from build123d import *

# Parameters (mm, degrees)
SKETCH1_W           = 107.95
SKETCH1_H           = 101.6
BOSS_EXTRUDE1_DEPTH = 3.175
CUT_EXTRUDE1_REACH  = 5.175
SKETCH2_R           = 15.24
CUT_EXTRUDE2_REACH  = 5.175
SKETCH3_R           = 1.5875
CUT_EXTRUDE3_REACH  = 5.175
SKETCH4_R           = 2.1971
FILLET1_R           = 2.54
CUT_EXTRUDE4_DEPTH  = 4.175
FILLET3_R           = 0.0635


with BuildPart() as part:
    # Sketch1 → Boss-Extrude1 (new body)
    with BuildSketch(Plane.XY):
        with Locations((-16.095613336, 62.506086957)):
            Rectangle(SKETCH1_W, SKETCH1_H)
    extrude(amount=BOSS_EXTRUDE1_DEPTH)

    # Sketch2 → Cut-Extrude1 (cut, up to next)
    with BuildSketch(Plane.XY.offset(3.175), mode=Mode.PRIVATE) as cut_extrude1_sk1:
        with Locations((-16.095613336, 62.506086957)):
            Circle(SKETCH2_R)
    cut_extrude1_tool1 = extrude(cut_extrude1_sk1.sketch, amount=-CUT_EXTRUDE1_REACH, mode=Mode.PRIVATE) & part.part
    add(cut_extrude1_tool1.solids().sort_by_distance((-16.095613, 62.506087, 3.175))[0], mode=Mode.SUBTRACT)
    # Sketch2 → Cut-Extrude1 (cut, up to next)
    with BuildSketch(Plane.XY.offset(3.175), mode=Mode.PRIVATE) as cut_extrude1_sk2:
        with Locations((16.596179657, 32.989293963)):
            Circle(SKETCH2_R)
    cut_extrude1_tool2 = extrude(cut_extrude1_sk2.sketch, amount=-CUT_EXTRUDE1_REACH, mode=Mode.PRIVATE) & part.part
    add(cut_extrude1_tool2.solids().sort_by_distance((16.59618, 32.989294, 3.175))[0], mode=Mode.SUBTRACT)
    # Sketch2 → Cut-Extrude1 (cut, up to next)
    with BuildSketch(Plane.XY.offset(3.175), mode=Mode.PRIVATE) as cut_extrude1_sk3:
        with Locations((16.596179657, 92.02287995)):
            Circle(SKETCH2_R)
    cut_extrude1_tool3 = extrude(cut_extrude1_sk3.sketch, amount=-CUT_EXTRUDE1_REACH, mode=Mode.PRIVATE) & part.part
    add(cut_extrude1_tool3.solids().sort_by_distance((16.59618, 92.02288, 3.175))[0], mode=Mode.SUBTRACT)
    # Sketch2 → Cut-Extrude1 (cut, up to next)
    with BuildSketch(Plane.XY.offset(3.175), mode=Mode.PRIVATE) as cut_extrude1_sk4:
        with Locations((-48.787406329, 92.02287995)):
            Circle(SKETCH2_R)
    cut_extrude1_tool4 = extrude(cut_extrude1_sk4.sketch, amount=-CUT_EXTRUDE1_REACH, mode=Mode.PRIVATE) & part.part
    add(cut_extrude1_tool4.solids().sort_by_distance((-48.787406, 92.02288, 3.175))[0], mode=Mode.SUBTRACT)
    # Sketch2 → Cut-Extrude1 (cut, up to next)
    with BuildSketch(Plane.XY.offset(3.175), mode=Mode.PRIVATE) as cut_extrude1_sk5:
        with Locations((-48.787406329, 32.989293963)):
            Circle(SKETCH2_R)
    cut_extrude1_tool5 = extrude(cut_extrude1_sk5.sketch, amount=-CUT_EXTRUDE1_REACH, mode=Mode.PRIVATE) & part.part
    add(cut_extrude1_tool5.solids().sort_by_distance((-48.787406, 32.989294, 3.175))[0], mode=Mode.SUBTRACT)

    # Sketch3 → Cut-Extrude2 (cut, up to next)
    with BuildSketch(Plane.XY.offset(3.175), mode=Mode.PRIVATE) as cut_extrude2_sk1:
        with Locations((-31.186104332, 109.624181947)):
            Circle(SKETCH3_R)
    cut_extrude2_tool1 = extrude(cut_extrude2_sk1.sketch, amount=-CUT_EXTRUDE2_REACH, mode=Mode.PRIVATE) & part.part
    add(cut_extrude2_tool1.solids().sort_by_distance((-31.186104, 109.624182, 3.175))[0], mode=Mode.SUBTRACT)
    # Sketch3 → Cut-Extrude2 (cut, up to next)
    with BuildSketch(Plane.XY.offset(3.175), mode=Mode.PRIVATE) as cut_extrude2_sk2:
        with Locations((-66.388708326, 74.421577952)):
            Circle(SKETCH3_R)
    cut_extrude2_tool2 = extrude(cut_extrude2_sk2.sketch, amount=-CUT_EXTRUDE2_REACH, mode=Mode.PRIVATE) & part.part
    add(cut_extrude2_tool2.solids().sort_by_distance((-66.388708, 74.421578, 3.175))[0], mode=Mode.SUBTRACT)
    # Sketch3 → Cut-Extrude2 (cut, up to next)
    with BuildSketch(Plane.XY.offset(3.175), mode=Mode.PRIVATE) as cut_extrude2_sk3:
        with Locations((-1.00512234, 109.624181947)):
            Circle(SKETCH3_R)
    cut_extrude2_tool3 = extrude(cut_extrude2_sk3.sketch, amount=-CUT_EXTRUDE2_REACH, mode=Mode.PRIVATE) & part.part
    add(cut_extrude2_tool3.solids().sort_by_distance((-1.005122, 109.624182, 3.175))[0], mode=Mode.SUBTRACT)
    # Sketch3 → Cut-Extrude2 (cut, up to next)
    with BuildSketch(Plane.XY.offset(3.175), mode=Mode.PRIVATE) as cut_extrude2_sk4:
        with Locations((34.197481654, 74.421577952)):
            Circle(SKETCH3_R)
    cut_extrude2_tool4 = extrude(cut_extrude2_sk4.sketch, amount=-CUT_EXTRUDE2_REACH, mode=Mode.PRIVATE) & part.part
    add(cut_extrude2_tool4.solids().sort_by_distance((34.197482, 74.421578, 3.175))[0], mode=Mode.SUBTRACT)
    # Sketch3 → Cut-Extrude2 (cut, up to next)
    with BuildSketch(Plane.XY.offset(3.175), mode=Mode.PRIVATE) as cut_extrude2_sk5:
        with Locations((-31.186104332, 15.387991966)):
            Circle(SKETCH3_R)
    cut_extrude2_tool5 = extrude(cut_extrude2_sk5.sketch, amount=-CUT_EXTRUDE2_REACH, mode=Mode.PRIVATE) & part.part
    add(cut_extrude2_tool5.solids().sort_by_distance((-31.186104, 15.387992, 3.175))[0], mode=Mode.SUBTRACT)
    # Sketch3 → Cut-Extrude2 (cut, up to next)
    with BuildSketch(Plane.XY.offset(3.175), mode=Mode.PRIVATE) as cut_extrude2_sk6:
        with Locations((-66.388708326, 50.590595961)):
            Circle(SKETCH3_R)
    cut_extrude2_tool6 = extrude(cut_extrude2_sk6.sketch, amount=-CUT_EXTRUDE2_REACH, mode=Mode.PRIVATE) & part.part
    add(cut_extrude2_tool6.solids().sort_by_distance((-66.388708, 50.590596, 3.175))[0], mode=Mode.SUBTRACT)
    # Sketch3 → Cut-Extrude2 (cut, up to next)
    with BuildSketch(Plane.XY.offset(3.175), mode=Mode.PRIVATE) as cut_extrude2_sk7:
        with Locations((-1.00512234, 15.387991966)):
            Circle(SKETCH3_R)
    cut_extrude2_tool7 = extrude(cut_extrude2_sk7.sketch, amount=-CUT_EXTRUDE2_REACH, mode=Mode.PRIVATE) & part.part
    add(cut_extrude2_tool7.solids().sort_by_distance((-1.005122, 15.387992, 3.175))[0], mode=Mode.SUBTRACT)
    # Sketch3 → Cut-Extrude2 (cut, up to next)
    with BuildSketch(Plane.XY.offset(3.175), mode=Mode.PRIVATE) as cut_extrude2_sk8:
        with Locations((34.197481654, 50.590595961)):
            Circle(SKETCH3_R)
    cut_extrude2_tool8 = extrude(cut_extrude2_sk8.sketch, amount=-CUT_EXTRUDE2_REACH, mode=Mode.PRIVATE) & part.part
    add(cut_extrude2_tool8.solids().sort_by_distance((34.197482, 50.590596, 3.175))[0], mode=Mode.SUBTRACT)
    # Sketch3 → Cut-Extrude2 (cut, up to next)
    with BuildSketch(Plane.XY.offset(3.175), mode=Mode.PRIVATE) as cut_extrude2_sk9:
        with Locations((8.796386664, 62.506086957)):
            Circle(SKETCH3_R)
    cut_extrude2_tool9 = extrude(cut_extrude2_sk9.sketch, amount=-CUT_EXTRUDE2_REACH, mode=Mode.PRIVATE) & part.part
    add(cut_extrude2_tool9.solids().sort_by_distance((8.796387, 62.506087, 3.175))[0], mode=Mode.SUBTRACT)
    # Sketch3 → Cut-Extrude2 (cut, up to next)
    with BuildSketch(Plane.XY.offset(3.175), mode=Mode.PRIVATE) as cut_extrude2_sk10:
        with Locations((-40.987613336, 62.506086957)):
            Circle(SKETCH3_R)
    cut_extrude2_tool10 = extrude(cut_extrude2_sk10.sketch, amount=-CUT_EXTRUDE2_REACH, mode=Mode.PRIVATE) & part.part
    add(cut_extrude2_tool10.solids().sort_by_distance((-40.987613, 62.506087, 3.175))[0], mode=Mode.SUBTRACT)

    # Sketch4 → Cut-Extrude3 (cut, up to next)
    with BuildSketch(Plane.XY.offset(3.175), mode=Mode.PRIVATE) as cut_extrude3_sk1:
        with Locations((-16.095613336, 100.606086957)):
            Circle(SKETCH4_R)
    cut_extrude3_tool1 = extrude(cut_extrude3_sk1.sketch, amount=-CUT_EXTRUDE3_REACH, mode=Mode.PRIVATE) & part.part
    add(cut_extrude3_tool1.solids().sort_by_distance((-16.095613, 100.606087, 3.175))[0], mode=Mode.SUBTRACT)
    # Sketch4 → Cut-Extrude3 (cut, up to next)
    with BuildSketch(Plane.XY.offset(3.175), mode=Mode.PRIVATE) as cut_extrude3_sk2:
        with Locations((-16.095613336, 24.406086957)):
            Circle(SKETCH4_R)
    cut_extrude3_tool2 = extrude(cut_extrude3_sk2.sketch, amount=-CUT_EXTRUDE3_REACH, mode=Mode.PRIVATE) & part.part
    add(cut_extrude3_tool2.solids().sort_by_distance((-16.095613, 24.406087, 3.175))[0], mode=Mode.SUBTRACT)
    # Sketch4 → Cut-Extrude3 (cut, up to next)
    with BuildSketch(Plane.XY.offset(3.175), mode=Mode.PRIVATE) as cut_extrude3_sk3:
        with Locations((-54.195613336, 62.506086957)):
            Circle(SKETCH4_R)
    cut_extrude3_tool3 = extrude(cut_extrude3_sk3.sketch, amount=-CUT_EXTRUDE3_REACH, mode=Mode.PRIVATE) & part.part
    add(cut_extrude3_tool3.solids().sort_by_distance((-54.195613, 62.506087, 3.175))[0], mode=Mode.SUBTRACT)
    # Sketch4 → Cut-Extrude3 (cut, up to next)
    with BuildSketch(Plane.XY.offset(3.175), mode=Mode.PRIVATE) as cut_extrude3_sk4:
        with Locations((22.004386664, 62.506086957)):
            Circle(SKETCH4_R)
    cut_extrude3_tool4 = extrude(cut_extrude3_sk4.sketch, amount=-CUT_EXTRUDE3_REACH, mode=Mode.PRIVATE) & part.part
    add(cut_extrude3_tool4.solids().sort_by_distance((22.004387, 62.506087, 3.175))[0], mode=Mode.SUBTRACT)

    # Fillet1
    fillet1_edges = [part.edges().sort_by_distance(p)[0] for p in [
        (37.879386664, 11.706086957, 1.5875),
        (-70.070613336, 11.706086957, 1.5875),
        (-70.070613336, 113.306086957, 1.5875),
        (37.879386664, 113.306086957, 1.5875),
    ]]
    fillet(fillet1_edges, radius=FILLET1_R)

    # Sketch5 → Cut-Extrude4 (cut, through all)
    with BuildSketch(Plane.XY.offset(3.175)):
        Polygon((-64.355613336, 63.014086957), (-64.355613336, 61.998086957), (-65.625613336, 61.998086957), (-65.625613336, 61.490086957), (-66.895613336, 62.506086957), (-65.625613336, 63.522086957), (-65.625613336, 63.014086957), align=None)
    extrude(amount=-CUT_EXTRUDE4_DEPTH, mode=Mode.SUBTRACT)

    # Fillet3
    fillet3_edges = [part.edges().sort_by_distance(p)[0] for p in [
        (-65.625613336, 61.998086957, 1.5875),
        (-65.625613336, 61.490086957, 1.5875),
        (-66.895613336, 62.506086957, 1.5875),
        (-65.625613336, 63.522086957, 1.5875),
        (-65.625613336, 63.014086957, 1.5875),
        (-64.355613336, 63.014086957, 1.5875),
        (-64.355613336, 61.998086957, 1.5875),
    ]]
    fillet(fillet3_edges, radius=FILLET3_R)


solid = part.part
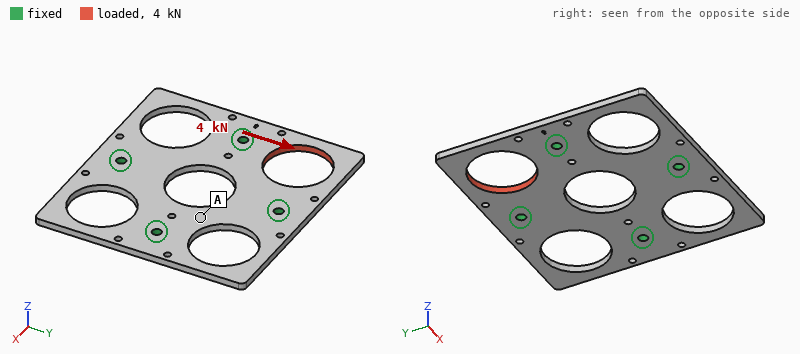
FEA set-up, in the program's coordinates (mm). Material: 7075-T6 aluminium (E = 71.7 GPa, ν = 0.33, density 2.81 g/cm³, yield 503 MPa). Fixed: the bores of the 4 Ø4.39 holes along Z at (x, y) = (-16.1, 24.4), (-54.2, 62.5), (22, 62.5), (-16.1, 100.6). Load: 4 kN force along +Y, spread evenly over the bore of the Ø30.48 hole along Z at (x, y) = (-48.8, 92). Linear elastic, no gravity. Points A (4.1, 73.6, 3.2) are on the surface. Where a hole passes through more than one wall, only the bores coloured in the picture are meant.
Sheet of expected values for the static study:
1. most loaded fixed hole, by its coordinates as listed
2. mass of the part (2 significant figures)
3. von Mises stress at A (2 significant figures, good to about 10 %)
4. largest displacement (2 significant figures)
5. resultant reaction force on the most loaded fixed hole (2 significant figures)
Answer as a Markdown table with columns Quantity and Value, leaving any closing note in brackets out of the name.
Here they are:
| Quantity | Value |
|---|---|
| most loaded fixed hole, by its coordinates as listed | (-54.2, 62.5) |
| mass of the part | 64 g |
| von Mises stress at A | 13 MPa |
| largest displacement | 68 µm |
| resultant reaction force on the most loaded fixed hole | 2.5 kN |
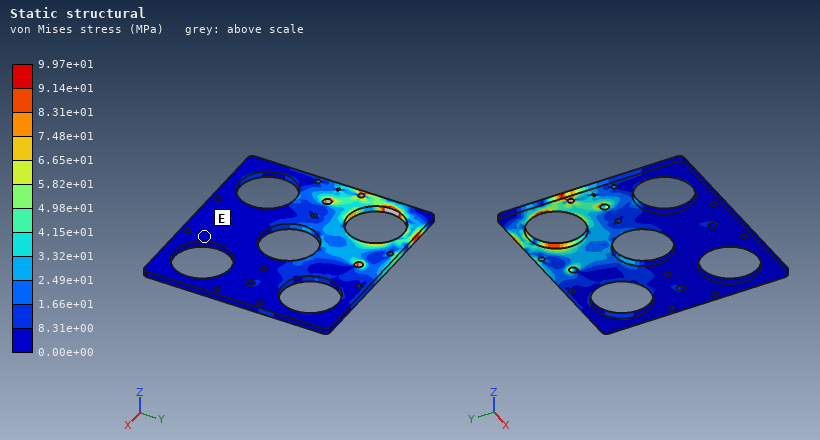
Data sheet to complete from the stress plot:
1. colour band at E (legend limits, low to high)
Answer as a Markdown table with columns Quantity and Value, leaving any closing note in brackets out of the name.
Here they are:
| Quantity | Value |
|---|---|
| colour band at E | 0.00e+00 to 8.31e+00 MPa |
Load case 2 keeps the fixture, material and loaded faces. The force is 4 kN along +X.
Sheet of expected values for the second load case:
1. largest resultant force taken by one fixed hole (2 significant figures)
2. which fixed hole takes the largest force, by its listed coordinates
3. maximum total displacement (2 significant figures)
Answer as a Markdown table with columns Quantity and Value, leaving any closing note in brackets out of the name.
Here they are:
| Quantity | Value |
|---|---|
| largest resultant force taken by one fixed hole | 2.4 kN |
| which fixed hole takes the largest force, by its listed coordinates | (-16.1, 100.6) |
| maximum total displacement | 64 µm |
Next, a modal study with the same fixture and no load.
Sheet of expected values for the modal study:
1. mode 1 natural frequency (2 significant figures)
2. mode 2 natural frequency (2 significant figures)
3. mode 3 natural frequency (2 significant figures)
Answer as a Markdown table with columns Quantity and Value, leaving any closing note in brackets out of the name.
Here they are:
| Quantity | Value |
|---|---|
| mode 1 natural frequency | 1600 Hz |
| mode 2 natural frequency | 1700 Hz |
| mode 3 natural frequency | 1700 Hz |
